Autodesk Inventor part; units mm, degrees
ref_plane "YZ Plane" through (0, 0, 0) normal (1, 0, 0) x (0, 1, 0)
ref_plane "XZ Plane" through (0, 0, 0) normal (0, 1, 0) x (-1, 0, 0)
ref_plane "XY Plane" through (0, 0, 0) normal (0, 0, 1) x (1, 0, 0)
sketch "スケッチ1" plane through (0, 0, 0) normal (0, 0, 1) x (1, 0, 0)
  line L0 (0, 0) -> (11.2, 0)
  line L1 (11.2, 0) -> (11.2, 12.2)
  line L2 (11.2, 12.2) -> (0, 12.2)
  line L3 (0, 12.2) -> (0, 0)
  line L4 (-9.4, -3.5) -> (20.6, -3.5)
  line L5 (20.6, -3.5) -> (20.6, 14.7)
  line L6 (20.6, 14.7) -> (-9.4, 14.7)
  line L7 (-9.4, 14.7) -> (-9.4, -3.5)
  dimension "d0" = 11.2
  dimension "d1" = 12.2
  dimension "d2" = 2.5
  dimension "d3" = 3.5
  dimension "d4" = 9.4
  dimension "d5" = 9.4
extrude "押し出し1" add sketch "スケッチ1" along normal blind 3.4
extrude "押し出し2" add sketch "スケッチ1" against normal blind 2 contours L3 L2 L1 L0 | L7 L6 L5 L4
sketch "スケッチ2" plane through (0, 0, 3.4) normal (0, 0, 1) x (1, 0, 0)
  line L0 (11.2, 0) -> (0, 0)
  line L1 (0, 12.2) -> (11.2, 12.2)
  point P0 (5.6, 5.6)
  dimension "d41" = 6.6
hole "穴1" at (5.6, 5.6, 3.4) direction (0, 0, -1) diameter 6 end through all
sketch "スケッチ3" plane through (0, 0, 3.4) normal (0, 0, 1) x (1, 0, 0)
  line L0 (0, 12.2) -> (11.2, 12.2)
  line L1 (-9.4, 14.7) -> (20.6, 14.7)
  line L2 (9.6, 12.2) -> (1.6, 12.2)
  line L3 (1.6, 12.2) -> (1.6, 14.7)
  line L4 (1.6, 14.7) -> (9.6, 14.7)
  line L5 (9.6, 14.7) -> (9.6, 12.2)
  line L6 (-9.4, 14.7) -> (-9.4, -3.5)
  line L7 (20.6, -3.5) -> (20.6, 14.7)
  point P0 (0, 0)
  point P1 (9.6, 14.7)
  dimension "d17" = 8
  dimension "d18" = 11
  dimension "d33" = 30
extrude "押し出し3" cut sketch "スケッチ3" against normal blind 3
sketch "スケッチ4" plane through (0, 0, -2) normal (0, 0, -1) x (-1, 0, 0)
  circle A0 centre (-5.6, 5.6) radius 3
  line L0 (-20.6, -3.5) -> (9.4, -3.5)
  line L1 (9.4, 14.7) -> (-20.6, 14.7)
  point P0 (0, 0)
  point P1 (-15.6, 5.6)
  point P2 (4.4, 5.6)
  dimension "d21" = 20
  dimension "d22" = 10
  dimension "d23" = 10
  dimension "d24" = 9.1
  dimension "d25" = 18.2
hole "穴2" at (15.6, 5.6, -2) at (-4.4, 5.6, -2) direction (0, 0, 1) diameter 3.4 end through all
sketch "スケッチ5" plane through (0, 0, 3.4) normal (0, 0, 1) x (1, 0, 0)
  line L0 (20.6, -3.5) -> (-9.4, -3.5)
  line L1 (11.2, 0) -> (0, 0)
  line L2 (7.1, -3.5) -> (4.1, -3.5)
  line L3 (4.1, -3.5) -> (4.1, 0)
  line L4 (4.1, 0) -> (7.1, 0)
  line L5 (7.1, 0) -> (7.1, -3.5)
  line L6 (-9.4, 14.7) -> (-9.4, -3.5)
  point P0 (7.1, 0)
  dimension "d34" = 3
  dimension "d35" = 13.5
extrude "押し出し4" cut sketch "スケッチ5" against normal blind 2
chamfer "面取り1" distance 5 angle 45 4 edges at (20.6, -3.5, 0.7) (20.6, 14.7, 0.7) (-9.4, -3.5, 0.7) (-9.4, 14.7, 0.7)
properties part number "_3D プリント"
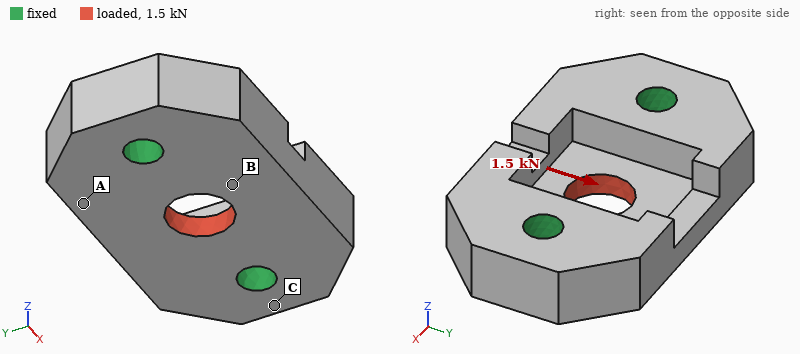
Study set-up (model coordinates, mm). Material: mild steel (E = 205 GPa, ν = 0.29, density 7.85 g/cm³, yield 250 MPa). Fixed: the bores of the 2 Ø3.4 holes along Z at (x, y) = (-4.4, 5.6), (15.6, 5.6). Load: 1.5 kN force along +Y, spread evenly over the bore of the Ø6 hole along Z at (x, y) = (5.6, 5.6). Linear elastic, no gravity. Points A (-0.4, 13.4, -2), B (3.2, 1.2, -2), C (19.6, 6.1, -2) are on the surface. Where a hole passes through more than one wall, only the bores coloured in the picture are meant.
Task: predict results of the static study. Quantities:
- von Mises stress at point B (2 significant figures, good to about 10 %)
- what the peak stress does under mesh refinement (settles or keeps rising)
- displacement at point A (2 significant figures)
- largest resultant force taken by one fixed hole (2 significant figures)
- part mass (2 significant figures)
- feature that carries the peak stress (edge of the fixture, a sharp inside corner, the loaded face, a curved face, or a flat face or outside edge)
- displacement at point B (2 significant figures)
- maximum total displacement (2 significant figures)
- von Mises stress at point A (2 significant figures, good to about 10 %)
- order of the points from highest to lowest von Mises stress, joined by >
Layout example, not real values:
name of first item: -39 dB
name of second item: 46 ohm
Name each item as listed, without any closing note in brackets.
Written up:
von Mises stress at point B: 40 MPa
what the peak stress does under mesh refinement: keeps rising
displacement at point A: 1.6 µm
largest resultant force taken by one fixed hole: 750 N
part mass: 16 g
feature that carries the peak stress: edge of the fixture
displacement at point B: 2.2 µm
maximum total displacement: 2.9 µm
von Mises stress at point A: 18 MPa
order of the points from highest to lowest von Mises stress, joined by >: B > A > C
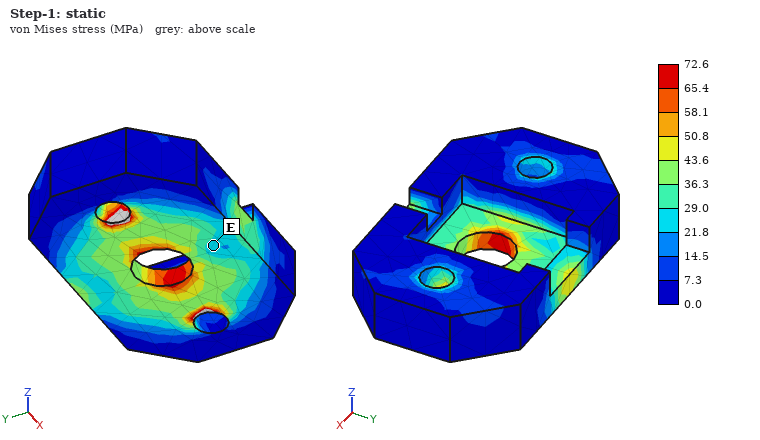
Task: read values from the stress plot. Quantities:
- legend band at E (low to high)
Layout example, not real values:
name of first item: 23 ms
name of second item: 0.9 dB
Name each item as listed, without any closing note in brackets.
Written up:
legend band at E: 21.8 to 29.0 MPa
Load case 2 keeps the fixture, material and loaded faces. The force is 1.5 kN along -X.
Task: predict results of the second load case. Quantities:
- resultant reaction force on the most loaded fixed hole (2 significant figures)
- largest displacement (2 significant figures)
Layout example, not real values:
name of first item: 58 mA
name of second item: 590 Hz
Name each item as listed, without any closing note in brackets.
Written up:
resultant reaction force on the most loaded fixed hole: 750 N
largest displacement: 1.6 µm
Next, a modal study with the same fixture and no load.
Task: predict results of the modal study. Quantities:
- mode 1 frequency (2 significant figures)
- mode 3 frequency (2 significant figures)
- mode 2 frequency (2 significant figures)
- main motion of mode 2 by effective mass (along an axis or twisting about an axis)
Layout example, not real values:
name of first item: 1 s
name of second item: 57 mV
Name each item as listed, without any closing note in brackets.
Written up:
mode 1 frequency: 36 kHz
mode 3 frequency: 52 kHz
mode 2 frequency: 40 kHz
main motion of mode 2 by effective mass: along Z
